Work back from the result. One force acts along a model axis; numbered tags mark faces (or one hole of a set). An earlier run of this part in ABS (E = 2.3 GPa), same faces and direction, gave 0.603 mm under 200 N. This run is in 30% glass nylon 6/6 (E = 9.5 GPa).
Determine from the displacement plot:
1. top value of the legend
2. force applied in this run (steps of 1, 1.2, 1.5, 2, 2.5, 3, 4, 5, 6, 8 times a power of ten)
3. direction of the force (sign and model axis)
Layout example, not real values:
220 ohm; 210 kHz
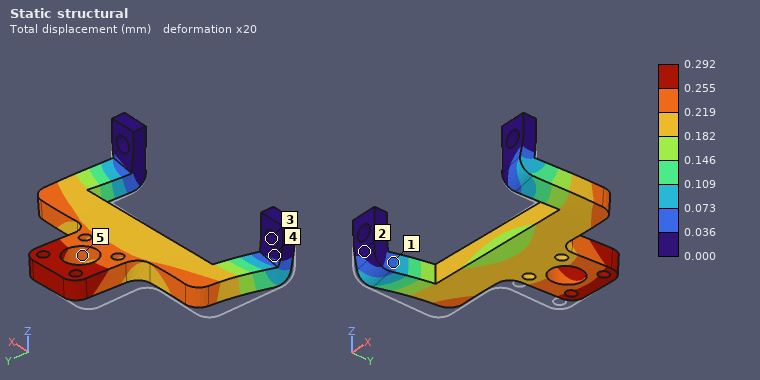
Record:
0.292 mm; 400 N; +X
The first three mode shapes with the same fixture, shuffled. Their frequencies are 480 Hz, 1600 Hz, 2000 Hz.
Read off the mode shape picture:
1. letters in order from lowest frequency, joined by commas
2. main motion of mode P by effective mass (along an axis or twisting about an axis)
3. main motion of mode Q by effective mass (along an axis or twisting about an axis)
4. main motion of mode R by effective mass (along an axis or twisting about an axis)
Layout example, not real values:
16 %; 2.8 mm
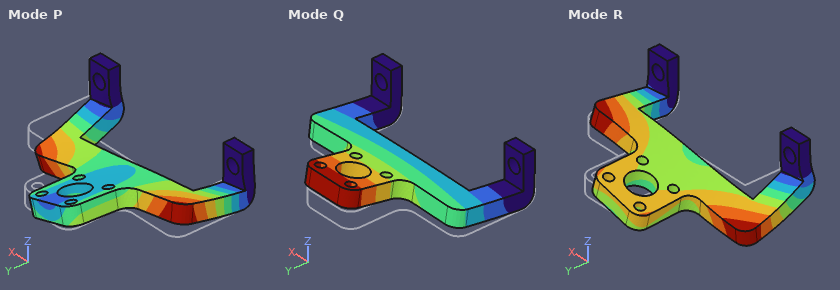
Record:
Q, R, P; along X; along Z; along X
